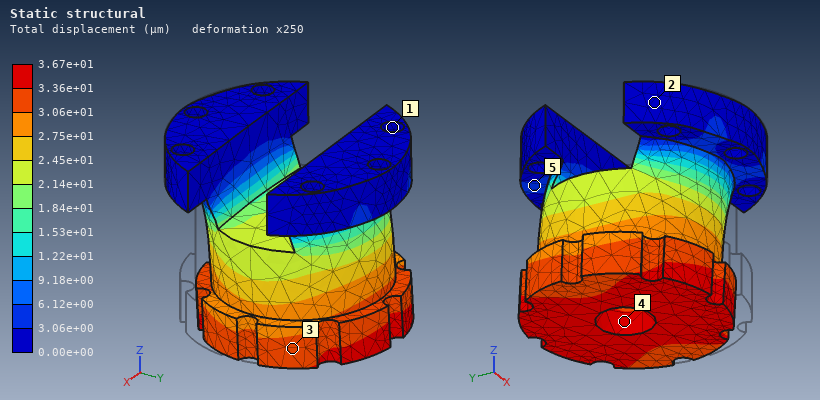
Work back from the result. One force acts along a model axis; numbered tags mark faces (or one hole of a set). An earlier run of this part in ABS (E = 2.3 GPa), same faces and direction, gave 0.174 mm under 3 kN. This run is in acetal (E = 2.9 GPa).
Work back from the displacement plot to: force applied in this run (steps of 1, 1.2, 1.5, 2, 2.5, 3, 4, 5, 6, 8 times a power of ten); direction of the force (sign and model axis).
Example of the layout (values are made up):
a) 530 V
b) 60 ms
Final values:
a) 800 N
b) +Y
